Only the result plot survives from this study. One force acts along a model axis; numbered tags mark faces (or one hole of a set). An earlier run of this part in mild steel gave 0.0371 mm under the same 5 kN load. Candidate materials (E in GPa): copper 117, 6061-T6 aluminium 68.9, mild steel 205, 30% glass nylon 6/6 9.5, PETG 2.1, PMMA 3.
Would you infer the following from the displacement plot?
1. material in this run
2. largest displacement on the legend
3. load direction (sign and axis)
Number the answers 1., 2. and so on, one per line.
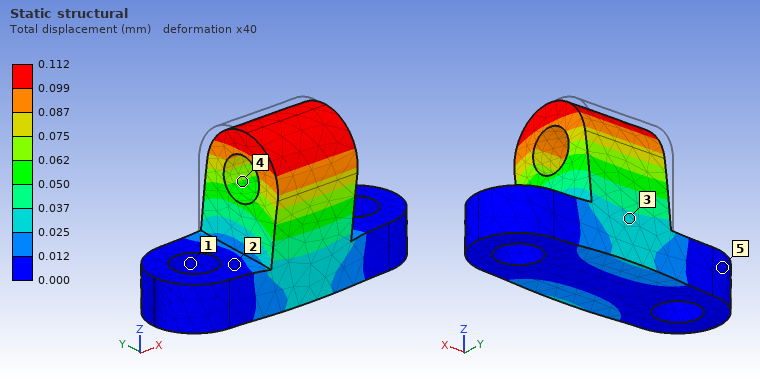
1. 6061-T6 aluminium
2. 0.112 mm
3. -Y
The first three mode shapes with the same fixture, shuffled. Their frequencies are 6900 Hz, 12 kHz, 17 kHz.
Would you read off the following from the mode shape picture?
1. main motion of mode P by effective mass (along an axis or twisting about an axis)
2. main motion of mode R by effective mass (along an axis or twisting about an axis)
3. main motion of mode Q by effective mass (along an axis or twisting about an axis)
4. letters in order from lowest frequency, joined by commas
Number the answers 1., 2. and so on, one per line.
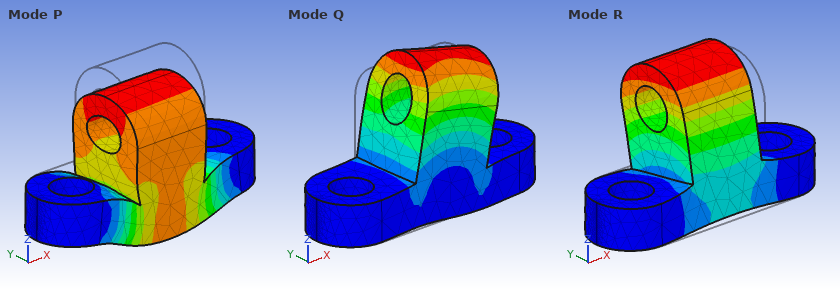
1. along Z
2. along Y
3. along X
4. R, Q, P
